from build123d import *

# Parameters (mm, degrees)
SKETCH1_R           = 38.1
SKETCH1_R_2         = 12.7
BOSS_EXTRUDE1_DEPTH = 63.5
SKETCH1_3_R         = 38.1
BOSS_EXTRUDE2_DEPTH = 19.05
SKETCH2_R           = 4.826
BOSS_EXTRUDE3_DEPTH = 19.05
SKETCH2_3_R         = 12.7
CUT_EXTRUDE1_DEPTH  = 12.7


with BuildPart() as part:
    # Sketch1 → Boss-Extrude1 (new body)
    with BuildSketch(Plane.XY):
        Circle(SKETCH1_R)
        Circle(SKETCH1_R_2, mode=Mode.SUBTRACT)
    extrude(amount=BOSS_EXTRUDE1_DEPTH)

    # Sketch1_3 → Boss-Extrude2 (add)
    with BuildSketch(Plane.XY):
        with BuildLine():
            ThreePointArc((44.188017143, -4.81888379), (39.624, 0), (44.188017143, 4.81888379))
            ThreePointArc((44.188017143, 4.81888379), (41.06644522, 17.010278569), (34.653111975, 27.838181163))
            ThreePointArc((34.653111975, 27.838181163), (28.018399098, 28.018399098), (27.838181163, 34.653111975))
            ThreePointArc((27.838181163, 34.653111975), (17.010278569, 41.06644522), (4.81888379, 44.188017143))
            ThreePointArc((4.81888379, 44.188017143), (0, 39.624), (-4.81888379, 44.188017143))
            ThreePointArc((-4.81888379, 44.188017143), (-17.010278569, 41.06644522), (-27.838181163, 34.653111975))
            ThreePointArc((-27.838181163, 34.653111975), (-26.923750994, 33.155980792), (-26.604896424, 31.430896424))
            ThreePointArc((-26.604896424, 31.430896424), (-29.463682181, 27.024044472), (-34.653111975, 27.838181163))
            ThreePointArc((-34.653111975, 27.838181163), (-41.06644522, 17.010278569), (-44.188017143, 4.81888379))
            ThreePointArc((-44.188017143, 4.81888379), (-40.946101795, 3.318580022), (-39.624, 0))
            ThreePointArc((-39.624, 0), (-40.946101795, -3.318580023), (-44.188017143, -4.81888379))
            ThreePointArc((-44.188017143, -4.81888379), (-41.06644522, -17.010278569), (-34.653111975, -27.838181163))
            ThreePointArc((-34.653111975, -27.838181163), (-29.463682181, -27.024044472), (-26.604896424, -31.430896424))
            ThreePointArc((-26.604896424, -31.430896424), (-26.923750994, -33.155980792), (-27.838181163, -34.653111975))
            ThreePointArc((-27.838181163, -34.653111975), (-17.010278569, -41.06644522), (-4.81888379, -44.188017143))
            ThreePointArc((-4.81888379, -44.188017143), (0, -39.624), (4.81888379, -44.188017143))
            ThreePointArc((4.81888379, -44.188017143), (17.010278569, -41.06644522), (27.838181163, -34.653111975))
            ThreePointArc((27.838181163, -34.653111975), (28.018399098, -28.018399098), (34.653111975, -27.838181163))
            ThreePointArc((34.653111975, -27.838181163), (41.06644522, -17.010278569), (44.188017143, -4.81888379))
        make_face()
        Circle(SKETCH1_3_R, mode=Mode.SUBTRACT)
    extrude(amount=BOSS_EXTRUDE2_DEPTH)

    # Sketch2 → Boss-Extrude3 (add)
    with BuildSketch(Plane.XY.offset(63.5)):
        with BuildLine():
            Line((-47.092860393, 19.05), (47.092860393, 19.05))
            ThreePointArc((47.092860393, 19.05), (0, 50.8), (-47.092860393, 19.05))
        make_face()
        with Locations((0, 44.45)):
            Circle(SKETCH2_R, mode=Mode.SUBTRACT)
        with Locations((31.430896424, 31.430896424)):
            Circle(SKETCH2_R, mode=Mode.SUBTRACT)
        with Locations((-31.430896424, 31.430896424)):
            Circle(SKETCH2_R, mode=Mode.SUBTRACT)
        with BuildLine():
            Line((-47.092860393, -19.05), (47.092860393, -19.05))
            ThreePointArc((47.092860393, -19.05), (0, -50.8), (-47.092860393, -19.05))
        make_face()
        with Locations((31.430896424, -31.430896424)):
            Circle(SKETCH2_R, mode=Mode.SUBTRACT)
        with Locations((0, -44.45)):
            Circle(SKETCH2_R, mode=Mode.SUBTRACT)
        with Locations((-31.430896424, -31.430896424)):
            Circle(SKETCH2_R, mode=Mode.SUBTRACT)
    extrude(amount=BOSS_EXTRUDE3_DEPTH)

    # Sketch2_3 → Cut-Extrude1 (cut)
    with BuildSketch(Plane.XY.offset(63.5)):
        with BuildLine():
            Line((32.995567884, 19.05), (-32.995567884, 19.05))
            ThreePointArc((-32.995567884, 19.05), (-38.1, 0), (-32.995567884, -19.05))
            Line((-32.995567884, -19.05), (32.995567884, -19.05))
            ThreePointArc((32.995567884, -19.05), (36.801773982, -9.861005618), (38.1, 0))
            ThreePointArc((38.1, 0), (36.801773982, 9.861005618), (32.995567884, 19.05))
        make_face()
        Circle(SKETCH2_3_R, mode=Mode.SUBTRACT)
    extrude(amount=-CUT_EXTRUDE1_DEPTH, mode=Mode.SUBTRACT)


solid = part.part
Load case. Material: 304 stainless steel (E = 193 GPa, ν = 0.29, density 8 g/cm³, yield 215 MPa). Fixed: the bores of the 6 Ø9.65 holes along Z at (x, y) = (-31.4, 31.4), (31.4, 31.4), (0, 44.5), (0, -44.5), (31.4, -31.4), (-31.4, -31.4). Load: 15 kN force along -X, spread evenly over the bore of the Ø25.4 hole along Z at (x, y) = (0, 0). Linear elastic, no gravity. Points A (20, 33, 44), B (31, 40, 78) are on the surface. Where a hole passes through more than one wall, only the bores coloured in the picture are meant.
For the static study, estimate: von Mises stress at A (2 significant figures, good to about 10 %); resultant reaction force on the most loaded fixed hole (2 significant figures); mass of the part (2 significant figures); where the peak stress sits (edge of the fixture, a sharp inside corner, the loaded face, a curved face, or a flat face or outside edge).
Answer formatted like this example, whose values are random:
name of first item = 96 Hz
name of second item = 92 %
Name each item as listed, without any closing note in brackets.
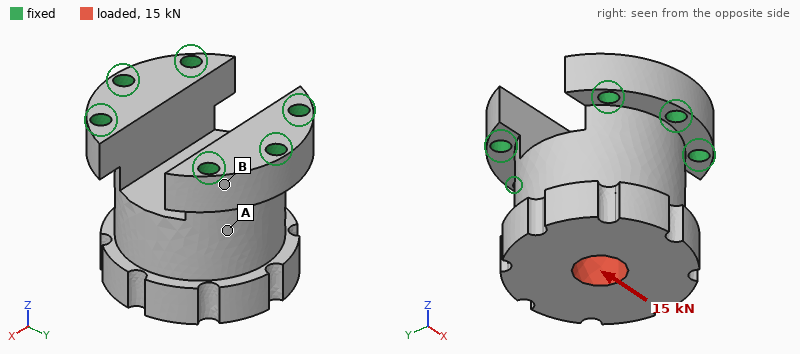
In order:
von Mises stress at A = 13 MPa
resultant reaction force on the most loaded fixed hole = 6.6 kN
mass of the part = 2.6 kg
where the peak stress sits = edge of the fixture
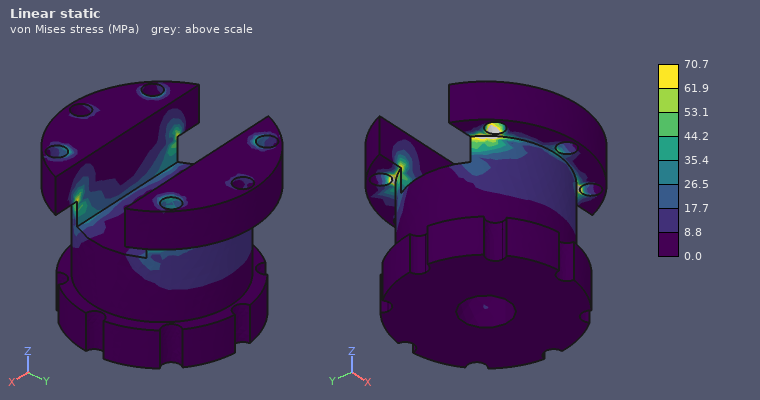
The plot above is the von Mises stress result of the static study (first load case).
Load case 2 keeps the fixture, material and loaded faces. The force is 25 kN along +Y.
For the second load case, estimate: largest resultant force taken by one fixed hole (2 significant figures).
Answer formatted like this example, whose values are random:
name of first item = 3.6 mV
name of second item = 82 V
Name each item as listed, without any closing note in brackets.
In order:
largest resultant force taken by one fixed hole = 12 kN
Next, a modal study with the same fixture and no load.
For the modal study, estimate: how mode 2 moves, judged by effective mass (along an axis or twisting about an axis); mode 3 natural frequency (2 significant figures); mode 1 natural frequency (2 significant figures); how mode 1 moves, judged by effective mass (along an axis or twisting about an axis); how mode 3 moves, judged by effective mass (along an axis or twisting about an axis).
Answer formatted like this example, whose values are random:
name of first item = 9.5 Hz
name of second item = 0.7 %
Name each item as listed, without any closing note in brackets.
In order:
how mode 2 moves, judged by effective mass = along Y
mode 3 natural frequency = 6700 Hz
mode 1 natural frequency = 3700 Hz
how mode 1 moves, judged by effective mass = along X
how mode 3 moves, judged by effective mass = twisting about Z
